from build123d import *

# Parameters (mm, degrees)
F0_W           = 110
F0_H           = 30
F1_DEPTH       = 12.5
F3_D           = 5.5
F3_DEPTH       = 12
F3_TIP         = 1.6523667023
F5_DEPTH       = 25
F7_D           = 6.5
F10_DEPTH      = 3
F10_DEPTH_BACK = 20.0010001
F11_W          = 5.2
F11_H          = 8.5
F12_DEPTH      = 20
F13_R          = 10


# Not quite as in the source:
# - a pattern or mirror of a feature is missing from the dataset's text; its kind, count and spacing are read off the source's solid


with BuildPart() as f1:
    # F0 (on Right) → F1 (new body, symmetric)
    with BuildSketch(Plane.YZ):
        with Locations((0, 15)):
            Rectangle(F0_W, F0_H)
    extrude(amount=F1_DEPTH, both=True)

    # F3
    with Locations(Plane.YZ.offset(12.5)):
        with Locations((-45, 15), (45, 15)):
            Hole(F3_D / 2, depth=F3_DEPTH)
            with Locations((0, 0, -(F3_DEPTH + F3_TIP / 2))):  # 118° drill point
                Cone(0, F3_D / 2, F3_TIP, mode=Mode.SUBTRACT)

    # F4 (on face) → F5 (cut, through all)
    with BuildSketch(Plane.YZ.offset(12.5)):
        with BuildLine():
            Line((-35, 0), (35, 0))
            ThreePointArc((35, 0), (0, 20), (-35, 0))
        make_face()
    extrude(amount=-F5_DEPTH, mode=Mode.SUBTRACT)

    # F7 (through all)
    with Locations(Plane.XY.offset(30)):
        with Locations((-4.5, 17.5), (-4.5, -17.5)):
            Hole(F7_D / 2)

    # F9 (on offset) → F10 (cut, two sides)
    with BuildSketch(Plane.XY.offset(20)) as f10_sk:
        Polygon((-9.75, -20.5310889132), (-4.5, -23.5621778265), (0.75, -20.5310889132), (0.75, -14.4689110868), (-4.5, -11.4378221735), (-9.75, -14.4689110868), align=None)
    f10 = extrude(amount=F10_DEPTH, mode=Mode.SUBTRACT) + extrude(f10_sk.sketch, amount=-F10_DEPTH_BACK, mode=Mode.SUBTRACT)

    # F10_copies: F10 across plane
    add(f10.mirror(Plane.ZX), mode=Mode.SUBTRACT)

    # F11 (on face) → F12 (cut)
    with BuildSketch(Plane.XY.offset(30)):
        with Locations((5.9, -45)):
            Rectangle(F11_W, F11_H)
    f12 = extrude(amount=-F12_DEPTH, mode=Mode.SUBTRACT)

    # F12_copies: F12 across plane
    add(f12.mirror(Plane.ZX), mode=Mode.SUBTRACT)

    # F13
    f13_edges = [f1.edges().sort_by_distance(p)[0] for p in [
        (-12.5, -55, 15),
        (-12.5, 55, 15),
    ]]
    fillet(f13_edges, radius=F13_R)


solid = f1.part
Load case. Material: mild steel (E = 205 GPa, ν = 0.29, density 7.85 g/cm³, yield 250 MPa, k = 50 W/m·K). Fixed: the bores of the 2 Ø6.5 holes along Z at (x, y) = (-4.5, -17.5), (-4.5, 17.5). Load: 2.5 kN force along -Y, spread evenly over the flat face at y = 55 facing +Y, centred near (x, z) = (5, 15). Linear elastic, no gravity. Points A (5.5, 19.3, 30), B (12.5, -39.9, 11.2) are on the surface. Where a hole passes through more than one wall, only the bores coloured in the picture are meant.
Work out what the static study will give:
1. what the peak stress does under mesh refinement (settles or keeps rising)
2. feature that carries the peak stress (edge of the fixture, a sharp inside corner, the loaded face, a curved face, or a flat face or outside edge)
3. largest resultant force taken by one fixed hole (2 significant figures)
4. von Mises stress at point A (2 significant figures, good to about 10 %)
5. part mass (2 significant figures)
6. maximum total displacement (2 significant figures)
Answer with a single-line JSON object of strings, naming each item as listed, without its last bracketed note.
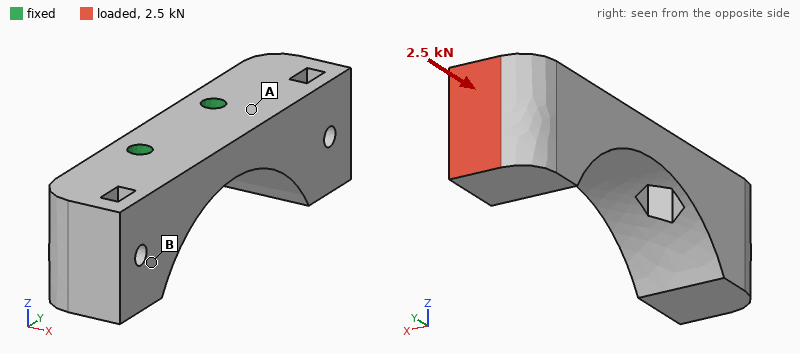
{"what the peak stress does under mesh refinement": "keeps rising", "feature that carries the peak stress": "edge of the fixture", "largest resultant force taken by one fixed hole": "1.5 kN", "von Mises stress at point A": "14 MPa", "part mass": "410 g", "maximum total displacement": "23 µm"}
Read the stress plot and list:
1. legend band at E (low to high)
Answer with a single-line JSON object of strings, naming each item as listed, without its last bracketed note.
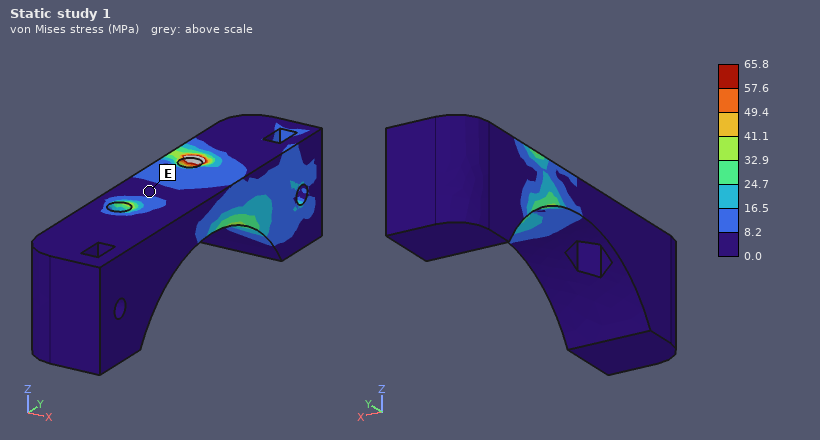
{"legend band at E": "0.0 to 8.2 MPa"}
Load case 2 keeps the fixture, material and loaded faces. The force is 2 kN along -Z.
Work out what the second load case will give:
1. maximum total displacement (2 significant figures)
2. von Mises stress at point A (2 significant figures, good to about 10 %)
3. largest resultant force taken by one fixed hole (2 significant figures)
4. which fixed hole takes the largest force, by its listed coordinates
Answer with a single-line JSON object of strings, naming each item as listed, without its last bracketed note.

{"maximum total displacement": "70 µm", "von Mises stress at point A": "74 MPa", "largest resultant force taken by one fixed hole": "3.4 kN", "which fixed hole takes the largest force, by its listed coordinates": "(-4.5, 17.5)"}
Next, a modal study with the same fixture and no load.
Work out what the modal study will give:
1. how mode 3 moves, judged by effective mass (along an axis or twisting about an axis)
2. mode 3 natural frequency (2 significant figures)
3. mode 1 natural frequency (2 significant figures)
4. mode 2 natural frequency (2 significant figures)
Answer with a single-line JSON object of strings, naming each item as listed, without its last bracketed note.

{"how mode 3 moves, judged by effective mass": "along X", "mode 3 natural frequency": "4800 Hz", "mode 1 natural frequency": "3400 Hz", "mode 2 natural frequency": "3600 Hz"}
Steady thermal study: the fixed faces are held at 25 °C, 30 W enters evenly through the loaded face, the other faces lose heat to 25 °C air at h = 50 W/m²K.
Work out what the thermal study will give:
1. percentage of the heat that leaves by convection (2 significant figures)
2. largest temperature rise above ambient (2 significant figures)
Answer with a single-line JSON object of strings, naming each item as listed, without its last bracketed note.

{"percentage of the heat that leaves by convection": "27 %", "largest temperature rise above ambient": "53 K"}
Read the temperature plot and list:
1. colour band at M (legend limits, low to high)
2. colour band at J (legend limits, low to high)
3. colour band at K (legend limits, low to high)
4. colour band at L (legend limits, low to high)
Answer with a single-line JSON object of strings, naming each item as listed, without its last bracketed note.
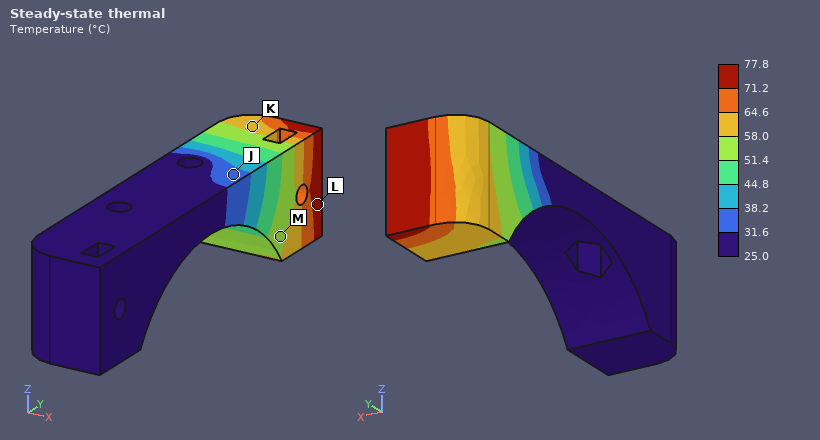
{"colour band at M": "51.4 to 58.0 °C", "colour band at J": "31.6 to 38.2 °C", "colour band at K": "58.0 to 64.6 °C", "colour band at L": "71.2 to 77.8 °C"}
